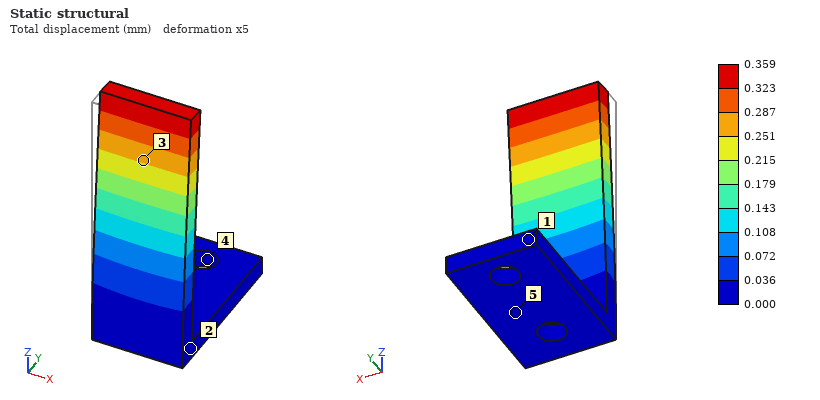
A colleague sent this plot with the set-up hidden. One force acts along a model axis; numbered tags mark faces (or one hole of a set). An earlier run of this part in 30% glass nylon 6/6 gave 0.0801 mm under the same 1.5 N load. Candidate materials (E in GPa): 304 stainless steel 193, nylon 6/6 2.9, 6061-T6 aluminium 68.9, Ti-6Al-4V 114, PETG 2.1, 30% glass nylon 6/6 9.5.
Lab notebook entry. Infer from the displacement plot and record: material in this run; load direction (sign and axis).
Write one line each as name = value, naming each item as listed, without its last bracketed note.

material in this run = PETG
load direction = +Y
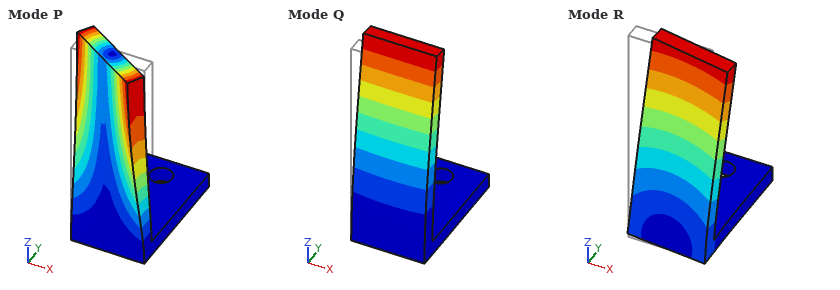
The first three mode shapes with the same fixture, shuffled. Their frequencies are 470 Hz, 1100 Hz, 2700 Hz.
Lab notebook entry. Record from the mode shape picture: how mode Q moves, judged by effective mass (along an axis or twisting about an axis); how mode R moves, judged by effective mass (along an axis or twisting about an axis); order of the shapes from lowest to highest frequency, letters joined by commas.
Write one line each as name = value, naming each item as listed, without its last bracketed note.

how mode Q moves, judged by effective mass = along Y
how mode R moves, judged by effective mass = along X
order of the shapes from lowest to highest frequency, letters joined by commas = Q, R, P
